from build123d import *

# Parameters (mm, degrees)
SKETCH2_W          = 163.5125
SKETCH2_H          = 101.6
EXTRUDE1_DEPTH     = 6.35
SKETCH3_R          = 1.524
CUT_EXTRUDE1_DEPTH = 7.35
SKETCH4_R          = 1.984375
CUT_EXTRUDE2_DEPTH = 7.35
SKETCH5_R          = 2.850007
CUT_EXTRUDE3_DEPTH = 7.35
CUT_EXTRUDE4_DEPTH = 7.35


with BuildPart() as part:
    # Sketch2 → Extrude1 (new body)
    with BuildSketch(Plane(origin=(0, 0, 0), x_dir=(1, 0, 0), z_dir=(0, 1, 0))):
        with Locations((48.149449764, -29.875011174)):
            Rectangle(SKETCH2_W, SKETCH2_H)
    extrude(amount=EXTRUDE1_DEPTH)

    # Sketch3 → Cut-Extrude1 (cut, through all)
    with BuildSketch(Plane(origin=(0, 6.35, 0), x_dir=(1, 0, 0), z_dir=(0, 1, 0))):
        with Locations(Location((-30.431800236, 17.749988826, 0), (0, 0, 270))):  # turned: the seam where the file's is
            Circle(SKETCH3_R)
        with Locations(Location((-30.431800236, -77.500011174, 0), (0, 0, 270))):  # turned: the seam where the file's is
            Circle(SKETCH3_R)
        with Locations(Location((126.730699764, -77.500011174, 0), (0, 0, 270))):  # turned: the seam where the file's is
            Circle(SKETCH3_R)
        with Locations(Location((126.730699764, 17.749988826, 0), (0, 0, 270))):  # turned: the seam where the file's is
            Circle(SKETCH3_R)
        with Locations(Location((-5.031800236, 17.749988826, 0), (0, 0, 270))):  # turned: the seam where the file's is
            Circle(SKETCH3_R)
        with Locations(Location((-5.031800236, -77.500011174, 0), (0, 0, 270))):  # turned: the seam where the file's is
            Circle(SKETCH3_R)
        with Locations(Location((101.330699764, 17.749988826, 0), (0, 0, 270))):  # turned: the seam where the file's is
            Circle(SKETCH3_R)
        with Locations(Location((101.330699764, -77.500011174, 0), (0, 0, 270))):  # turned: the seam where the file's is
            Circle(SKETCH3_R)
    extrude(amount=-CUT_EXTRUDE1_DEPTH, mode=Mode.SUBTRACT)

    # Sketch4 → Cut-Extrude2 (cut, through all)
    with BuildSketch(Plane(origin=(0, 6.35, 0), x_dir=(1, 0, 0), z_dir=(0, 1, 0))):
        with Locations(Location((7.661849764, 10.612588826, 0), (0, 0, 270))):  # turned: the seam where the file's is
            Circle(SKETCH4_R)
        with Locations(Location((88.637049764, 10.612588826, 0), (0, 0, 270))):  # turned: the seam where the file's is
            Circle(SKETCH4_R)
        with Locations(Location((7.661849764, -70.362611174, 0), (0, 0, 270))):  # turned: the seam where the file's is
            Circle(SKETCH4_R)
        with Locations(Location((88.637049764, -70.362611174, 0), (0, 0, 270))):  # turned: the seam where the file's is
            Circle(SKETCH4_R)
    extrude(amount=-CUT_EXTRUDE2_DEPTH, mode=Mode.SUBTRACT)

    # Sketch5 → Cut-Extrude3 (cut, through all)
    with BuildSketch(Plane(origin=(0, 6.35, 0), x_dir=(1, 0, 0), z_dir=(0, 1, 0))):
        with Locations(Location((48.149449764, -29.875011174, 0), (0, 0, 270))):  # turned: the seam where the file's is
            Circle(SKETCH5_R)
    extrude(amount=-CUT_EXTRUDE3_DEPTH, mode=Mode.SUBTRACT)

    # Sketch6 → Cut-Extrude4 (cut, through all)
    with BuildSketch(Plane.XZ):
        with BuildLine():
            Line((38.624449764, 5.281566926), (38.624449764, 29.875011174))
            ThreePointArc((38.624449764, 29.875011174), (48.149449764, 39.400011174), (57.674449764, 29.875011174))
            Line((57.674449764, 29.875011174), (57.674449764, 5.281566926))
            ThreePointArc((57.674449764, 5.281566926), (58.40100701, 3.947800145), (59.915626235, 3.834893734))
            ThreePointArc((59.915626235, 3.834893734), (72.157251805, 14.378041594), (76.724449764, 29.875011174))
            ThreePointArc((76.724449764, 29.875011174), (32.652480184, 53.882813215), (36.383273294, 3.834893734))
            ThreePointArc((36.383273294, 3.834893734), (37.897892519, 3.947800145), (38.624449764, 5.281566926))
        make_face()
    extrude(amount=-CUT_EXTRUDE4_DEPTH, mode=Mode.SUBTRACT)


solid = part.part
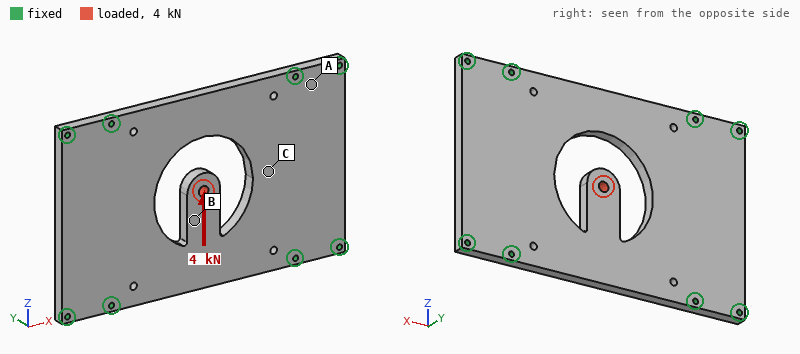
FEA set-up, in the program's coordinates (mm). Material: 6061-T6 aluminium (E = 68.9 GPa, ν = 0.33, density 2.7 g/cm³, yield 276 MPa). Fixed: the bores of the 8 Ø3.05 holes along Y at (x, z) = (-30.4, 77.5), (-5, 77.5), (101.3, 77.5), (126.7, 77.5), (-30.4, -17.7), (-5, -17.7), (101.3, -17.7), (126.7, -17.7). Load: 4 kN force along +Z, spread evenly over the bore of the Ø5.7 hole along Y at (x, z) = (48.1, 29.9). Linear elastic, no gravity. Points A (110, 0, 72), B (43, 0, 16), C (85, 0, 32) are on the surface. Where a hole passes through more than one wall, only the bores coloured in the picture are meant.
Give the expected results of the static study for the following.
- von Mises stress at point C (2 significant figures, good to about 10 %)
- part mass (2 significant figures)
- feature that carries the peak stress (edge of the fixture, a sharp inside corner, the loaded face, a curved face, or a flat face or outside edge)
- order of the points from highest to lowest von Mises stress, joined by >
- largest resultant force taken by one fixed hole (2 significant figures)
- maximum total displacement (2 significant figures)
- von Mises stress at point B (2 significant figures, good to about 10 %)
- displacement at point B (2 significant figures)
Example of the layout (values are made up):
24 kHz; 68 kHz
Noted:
12 MPa; 250 g; a curved face; B > C > A; 1.2 kN; 48 µm; 33 MPa; 37 µm
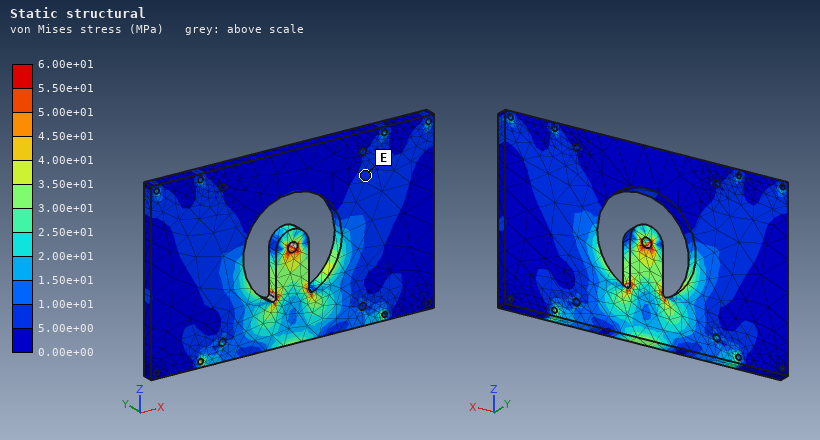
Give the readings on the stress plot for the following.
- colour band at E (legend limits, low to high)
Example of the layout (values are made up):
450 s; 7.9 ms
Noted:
5.00e+00 to 1.00e+01 MPa
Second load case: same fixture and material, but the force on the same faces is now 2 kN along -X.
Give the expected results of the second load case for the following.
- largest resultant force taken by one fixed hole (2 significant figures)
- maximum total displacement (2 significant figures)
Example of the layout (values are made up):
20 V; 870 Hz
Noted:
1.1 kN; 0.17 mm
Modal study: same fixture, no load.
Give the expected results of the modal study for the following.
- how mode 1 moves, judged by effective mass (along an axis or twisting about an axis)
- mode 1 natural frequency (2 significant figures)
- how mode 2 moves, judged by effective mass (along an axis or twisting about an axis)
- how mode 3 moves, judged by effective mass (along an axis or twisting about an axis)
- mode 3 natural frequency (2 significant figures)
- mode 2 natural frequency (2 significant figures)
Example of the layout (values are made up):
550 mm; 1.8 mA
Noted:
along Y; 1700 Hz; along Y; twisting about Z; 3200 Hz; 2700 Hz
